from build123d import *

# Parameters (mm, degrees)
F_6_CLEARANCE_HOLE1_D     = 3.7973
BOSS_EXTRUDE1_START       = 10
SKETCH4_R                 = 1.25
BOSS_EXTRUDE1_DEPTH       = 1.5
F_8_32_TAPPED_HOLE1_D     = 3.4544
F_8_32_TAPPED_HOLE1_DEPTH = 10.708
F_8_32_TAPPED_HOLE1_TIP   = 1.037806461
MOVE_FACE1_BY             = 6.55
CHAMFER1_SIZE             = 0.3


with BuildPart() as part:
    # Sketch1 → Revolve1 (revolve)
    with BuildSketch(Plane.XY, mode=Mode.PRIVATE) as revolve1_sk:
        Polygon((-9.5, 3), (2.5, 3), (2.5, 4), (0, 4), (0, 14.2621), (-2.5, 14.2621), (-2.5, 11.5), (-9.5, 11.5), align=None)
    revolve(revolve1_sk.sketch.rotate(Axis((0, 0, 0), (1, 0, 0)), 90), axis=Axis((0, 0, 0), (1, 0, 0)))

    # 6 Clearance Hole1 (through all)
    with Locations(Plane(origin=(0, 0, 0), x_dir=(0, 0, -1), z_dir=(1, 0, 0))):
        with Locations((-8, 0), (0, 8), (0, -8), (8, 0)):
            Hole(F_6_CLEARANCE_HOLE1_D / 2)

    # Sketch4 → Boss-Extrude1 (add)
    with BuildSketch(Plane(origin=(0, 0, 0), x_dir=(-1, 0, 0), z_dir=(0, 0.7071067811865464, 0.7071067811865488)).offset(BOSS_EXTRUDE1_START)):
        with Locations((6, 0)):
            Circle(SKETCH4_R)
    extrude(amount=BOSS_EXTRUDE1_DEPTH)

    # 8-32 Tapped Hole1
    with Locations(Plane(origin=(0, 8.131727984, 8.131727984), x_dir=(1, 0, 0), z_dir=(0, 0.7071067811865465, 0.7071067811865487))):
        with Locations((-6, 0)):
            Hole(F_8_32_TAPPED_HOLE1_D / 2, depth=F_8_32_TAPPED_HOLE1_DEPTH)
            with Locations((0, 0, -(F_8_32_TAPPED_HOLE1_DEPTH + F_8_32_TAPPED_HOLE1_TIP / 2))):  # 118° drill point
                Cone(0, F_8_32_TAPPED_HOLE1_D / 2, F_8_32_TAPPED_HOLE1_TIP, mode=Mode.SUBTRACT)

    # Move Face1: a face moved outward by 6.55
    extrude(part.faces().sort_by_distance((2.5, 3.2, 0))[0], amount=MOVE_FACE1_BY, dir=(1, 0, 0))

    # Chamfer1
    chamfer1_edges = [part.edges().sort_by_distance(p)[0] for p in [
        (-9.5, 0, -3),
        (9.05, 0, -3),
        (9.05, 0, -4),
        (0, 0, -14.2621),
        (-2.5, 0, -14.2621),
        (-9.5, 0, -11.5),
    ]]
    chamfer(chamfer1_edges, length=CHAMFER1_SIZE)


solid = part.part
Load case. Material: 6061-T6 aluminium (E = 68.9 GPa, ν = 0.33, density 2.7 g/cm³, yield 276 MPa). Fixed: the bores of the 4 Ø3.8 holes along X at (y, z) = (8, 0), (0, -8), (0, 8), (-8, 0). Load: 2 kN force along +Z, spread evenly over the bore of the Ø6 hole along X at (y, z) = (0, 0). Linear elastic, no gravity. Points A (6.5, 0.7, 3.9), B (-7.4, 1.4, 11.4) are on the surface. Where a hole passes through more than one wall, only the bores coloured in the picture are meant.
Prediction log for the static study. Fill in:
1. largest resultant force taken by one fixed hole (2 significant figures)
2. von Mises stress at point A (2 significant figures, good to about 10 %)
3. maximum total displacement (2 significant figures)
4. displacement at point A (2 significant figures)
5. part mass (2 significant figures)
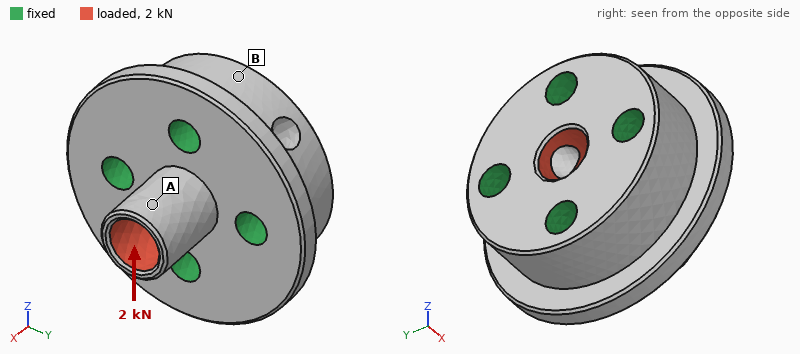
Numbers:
870 N
23 MPa
33 µm
27 µm
11 g
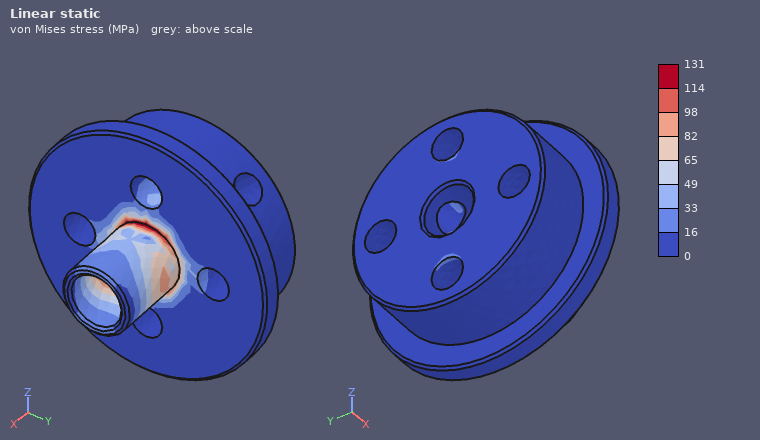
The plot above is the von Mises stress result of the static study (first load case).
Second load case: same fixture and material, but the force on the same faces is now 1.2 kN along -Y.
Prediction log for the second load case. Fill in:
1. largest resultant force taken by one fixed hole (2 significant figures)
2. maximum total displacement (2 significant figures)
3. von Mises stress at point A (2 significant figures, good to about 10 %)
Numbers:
520 N
20 µm
22 MPa
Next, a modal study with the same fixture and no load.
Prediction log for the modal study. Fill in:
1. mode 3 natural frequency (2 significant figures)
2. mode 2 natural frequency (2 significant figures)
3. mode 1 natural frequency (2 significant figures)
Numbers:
59 kHz
44 kHz
44 kHz
